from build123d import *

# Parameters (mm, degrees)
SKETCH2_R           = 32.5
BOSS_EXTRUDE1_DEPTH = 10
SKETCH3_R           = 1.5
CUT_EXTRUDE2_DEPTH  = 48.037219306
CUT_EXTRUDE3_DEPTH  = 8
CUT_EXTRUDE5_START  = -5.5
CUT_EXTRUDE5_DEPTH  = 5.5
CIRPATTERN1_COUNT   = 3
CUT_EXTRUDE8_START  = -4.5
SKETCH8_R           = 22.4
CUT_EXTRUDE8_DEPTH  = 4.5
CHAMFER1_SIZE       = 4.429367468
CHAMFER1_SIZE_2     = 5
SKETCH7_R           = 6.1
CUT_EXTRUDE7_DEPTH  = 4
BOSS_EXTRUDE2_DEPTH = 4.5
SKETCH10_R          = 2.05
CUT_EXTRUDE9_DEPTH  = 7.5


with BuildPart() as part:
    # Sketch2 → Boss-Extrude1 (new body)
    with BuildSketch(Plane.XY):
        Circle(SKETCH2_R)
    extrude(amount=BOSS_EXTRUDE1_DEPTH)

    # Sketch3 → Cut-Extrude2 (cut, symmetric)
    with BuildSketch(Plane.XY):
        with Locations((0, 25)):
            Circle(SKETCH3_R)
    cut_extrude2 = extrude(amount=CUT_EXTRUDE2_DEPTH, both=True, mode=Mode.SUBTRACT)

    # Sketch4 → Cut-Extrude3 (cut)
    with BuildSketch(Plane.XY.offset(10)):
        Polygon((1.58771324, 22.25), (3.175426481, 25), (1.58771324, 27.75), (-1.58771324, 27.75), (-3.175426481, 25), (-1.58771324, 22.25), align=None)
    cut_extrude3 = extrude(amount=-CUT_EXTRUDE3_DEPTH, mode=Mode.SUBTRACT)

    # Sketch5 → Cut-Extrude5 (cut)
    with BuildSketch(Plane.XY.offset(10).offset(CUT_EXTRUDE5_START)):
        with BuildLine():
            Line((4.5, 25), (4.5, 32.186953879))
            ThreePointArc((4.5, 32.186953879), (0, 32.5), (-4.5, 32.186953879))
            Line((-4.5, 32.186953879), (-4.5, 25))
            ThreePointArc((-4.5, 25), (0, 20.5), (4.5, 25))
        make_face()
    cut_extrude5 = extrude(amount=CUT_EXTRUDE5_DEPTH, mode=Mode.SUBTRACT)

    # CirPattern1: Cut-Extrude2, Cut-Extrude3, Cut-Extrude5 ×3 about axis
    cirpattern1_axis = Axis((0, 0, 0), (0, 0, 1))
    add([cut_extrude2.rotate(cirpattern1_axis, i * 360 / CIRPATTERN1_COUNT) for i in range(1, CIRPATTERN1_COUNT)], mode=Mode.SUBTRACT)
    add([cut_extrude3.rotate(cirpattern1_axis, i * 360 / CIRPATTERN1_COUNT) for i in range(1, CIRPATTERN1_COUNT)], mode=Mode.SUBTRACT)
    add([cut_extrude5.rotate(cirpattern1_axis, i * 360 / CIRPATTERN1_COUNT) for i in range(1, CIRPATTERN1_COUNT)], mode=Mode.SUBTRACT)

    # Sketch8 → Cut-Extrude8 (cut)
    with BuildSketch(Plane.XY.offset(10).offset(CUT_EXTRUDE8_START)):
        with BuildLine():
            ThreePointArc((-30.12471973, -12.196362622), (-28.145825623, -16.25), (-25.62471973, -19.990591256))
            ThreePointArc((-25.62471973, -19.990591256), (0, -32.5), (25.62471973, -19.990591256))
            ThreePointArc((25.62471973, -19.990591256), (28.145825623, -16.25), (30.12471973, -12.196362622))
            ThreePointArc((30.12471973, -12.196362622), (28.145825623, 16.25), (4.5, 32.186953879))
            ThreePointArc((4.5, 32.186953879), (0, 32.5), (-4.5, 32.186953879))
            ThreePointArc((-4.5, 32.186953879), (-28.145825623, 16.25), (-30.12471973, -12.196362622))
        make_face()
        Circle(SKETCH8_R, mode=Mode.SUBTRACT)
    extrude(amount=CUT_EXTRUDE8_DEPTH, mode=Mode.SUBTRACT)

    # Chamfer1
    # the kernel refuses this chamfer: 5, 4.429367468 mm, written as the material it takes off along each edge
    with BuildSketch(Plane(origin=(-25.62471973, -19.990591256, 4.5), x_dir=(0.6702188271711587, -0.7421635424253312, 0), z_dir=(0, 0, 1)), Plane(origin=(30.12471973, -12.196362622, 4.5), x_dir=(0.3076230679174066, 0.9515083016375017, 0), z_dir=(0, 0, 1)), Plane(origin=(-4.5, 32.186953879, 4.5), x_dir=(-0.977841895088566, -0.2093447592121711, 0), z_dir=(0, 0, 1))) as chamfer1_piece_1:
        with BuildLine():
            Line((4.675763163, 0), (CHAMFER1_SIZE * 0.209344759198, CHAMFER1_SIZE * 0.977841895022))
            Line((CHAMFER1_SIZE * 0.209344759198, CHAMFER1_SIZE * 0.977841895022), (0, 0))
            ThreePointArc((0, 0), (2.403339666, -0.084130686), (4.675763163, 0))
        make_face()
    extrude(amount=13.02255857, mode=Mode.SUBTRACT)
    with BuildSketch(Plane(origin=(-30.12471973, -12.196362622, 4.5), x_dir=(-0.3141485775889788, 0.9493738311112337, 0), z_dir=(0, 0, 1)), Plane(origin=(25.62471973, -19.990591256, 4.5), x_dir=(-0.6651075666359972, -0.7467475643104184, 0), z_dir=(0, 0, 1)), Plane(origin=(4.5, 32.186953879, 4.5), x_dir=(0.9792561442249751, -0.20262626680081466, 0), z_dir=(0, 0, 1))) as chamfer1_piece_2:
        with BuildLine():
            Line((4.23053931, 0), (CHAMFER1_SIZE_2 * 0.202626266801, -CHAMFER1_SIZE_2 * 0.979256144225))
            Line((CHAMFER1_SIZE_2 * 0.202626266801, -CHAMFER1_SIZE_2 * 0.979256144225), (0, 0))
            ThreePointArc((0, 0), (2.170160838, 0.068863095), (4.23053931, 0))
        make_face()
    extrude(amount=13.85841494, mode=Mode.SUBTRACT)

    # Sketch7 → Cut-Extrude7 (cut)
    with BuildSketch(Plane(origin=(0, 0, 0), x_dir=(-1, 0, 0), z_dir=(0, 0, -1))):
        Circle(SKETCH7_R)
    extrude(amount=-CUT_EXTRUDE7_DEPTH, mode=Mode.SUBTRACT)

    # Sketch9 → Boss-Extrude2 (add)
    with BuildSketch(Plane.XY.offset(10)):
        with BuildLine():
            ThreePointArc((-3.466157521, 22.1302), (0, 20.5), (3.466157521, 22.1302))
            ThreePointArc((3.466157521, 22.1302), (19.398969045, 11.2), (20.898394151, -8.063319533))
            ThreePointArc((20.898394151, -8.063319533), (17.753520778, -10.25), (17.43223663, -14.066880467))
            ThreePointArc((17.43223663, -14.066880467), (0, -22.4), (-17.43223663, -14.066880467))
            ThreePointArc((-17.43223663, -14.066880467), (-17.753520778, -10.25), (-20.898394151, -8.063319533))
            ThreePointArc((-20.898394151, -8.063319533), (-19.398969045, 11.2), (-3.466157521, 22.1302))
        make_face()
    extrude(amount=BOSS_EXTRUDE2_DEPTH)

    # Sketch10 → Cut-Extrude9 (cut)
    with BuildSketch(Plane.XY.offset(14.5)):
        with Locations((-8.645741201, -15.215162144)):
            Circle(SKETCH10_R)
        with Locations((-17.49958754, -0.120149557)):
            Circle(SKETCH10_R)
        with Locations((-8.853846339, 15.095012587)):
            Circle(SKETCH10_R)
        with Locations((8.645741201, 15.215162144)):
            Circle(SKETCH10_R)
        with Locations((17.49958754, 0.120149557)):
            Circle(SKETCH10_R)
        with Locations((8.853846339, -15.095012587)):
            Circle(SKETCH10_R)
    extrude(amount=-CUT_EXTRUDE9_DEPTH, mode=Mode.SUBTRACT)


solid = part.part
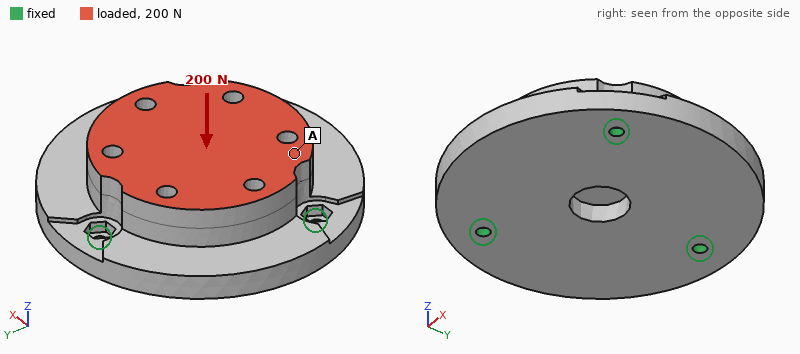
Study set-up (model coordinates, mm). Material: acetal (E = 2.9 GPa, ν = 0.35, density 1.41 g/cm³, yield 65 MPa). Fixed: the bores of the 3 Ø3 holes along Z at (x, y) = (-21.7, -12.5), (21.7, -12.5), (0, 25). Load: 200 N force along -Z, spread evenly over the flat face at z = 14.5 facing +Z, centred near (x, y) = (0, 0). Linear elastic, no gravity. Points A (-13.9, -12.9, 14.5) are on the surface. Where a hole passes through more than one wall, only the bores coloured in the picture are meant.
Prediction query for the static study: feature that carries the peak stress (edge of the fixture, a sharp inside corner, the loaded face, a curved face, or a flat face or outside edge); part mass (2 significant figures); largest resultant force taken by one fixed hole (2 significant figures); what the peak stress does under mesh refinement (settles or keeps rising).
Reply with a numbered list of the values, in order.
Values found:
1. edge of the fixture
2. 43 g
3. 78 N
4. keeps rising
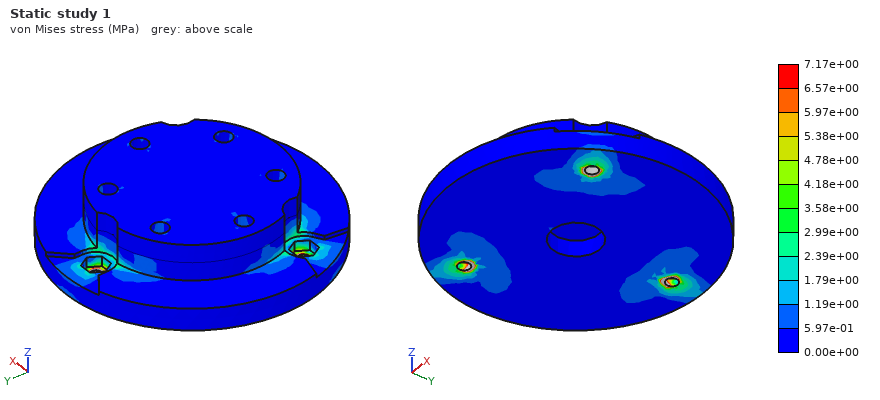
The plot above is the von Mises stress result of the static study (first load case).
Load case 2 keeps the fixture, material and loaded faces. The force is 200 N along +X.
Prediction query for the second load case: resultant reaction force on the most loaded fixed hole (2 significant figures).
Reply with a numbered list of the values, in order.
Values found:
1. 100 N
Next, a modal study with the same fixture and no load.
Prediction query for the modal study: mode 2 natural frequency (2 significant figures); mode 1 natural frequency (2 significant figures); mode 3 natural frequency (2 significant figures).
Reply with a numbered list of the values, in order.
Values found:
1. 2600 Hz
2. 2600 Hz
3. 2600 Hz
